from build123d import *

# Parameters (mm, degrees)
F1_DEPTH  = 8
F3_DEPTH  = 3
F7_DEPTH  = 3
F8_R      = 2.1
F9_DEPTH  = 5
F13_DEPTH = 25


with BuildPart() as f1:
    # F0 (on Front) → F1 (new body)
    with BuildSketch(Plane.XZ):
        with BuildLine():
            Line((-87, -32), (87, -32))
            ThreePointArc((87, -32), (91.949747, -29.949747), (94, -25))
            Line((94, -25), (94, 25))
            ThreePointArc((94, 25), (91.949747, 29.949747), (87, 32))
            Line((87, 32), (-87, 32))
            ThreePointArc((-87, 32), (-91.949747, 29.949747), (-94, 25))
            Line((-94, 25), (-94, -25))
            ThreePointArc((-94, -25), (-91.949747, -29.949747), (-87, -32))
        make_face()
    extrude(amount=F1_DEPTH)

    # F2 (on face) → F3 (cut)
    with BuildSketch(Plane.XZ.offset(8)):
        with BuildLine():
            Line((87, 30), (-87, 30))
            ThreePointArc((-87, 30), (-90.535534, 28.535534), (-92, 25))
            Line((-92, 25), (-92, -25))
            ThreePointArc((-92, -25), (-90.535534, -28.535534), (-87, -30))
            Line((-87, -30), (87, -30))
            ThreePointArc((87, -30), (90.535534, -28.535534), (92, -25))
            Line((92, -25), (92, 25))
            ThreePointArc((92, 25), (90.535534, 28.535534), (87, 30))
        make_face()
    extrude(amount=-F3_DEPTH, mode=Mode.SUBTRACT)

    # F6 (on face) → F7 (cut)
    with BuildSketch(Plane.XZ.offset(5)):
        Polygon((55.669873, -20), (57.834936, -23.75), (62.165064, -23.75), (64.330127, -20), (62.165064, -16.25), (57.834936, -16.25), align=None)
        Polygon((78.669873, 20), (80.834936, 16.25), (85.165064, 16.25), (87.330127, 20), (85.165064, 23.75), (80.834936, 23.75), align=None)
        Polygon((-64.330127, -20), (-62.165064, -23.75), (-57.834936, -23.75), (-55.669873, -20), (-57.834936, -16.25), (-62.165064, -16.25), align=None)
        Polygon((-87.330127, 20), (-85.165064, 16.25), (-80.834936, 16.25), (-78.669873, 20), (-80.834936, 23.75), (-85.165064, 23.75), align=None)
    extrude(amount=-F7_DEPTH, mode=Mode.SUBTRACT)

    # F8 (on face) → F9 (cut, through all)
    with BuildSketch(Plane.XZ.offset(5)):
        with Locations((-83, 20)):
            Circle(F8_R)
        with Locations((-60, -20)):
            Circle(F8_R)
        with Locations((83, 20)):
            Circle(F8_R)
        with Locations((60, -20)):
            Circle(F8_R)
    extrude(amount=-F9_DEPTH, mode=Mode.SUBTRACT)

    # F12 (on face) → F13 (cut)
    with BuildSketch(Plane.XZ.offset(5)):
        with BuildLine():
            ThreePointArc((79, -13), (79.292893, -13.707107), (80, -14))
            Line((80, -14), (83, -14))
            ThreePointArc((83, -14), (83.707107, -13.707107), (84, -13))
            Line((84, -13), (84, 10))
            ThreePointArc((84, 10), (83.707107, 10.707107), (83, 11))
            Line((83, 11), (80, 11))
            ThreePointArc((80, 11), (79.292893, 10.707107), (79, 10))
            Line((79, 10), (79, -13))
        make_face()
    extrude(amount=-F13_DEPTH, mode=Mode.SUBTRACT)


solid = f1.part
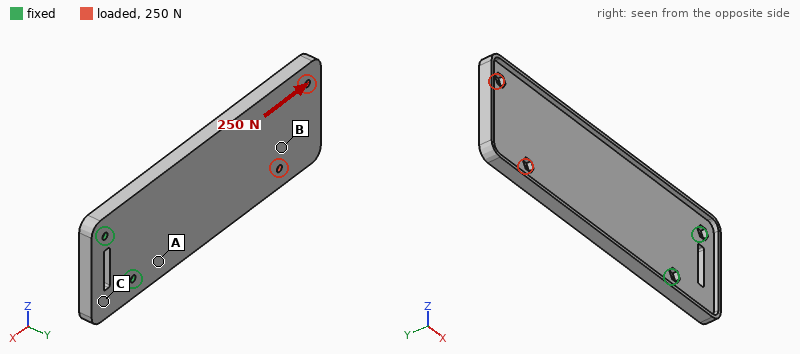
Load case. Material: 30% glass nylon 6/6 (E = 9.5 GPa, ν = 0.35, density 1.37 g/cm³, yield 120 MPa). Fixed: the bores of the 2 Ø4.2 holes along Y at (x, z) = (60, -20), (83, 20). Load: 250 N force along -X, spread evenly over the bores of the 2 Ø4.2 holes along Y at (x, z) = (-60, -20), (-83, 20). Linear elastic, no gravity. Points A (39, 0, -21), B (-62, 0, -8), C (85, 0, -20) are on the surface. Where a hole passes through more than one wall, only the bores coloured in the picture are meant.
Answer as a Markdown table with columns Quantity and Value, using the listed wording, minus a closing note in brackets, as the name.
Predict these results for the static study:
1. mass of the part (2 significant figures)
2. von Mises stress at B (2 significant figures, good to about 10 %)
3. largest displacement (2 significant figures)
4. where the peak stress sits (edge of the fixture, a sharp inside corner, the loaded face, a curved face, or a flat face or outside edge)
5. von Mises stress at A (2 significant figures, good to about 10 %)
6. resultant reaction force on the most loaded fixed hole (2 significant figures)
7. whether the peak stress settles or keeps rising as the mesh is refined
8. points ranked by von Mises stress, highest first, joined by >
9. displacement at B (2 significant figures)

| Quantity | Value |
|---|---|
| mass of the part | 84 g |
| von Mises stress at B | 1.3 MPa |
| largest displacement | 0.61 mm |
| where the peak stress sits | edge of the fixture |
| von Mises stress at A | 2.2 MPa |
| resultant reaction force on the most loaded fixed hole | 130 N |
| whether the peak stress settles or keeps rising as the mesh is refined | keeps rising |
| points ranked by von Mises stress, highest first, joined by > | A > B > C |
| displacement at B | 0.40 mm |
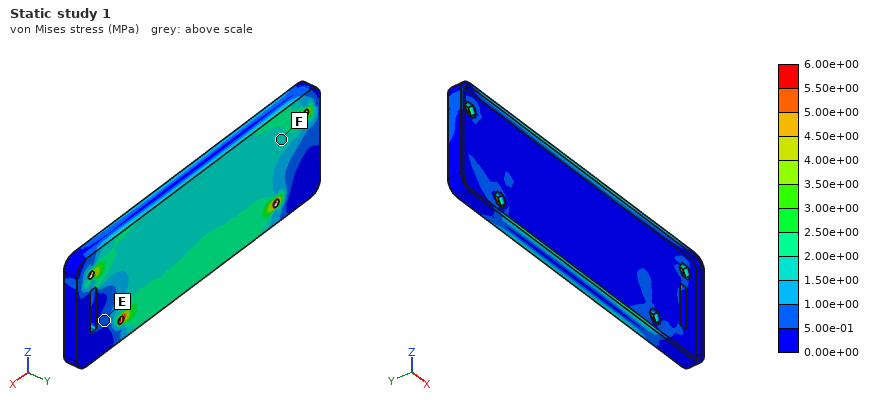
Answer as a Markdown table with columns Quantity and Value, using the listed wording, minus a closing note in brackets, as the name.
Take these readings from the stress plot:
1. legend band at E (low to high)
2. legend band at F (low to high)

| Quantity | Value |
|---|---|
| legend band at E | 5.00e-01 to 1.00e+00 MPa |
| legend band at F | 1.50e+00 to 2.00e+00 MPa |
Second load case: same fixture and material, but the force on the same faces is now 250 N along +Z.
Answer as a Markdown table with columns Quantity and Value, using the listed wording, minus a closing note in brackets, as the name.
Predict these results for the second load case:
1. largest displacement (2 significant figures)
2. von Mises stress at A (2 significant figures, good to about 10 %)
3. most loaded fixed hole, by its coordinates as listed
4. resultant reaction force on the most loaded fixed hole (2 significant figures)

| Quantity | Value |
|---|---|
| largest displacement | 0.64 mm |
| von Mises stress at A | 6.6 MPa |
| most loaded fixed hole, by its coordinates as listed | (60, -20) |
| resultant reaction force on the most loaded fixed hole | 820 N |
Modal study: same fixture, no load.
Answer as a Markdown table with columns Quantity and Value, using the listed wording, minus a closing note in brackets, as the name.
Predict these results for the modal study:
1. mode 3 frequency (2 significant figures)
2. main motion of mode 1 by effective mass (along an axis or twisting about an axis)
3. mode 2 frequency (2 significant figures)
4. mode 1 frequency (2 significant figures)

| Quantity | Value |
|---|---|
| mode 3 frequency | 500 Hz |
| main motion of mode 1 by effective mass | along Y |
| mode 2 frequency | 360 Hz |
| mode 1 frequency | 74 Hz |
